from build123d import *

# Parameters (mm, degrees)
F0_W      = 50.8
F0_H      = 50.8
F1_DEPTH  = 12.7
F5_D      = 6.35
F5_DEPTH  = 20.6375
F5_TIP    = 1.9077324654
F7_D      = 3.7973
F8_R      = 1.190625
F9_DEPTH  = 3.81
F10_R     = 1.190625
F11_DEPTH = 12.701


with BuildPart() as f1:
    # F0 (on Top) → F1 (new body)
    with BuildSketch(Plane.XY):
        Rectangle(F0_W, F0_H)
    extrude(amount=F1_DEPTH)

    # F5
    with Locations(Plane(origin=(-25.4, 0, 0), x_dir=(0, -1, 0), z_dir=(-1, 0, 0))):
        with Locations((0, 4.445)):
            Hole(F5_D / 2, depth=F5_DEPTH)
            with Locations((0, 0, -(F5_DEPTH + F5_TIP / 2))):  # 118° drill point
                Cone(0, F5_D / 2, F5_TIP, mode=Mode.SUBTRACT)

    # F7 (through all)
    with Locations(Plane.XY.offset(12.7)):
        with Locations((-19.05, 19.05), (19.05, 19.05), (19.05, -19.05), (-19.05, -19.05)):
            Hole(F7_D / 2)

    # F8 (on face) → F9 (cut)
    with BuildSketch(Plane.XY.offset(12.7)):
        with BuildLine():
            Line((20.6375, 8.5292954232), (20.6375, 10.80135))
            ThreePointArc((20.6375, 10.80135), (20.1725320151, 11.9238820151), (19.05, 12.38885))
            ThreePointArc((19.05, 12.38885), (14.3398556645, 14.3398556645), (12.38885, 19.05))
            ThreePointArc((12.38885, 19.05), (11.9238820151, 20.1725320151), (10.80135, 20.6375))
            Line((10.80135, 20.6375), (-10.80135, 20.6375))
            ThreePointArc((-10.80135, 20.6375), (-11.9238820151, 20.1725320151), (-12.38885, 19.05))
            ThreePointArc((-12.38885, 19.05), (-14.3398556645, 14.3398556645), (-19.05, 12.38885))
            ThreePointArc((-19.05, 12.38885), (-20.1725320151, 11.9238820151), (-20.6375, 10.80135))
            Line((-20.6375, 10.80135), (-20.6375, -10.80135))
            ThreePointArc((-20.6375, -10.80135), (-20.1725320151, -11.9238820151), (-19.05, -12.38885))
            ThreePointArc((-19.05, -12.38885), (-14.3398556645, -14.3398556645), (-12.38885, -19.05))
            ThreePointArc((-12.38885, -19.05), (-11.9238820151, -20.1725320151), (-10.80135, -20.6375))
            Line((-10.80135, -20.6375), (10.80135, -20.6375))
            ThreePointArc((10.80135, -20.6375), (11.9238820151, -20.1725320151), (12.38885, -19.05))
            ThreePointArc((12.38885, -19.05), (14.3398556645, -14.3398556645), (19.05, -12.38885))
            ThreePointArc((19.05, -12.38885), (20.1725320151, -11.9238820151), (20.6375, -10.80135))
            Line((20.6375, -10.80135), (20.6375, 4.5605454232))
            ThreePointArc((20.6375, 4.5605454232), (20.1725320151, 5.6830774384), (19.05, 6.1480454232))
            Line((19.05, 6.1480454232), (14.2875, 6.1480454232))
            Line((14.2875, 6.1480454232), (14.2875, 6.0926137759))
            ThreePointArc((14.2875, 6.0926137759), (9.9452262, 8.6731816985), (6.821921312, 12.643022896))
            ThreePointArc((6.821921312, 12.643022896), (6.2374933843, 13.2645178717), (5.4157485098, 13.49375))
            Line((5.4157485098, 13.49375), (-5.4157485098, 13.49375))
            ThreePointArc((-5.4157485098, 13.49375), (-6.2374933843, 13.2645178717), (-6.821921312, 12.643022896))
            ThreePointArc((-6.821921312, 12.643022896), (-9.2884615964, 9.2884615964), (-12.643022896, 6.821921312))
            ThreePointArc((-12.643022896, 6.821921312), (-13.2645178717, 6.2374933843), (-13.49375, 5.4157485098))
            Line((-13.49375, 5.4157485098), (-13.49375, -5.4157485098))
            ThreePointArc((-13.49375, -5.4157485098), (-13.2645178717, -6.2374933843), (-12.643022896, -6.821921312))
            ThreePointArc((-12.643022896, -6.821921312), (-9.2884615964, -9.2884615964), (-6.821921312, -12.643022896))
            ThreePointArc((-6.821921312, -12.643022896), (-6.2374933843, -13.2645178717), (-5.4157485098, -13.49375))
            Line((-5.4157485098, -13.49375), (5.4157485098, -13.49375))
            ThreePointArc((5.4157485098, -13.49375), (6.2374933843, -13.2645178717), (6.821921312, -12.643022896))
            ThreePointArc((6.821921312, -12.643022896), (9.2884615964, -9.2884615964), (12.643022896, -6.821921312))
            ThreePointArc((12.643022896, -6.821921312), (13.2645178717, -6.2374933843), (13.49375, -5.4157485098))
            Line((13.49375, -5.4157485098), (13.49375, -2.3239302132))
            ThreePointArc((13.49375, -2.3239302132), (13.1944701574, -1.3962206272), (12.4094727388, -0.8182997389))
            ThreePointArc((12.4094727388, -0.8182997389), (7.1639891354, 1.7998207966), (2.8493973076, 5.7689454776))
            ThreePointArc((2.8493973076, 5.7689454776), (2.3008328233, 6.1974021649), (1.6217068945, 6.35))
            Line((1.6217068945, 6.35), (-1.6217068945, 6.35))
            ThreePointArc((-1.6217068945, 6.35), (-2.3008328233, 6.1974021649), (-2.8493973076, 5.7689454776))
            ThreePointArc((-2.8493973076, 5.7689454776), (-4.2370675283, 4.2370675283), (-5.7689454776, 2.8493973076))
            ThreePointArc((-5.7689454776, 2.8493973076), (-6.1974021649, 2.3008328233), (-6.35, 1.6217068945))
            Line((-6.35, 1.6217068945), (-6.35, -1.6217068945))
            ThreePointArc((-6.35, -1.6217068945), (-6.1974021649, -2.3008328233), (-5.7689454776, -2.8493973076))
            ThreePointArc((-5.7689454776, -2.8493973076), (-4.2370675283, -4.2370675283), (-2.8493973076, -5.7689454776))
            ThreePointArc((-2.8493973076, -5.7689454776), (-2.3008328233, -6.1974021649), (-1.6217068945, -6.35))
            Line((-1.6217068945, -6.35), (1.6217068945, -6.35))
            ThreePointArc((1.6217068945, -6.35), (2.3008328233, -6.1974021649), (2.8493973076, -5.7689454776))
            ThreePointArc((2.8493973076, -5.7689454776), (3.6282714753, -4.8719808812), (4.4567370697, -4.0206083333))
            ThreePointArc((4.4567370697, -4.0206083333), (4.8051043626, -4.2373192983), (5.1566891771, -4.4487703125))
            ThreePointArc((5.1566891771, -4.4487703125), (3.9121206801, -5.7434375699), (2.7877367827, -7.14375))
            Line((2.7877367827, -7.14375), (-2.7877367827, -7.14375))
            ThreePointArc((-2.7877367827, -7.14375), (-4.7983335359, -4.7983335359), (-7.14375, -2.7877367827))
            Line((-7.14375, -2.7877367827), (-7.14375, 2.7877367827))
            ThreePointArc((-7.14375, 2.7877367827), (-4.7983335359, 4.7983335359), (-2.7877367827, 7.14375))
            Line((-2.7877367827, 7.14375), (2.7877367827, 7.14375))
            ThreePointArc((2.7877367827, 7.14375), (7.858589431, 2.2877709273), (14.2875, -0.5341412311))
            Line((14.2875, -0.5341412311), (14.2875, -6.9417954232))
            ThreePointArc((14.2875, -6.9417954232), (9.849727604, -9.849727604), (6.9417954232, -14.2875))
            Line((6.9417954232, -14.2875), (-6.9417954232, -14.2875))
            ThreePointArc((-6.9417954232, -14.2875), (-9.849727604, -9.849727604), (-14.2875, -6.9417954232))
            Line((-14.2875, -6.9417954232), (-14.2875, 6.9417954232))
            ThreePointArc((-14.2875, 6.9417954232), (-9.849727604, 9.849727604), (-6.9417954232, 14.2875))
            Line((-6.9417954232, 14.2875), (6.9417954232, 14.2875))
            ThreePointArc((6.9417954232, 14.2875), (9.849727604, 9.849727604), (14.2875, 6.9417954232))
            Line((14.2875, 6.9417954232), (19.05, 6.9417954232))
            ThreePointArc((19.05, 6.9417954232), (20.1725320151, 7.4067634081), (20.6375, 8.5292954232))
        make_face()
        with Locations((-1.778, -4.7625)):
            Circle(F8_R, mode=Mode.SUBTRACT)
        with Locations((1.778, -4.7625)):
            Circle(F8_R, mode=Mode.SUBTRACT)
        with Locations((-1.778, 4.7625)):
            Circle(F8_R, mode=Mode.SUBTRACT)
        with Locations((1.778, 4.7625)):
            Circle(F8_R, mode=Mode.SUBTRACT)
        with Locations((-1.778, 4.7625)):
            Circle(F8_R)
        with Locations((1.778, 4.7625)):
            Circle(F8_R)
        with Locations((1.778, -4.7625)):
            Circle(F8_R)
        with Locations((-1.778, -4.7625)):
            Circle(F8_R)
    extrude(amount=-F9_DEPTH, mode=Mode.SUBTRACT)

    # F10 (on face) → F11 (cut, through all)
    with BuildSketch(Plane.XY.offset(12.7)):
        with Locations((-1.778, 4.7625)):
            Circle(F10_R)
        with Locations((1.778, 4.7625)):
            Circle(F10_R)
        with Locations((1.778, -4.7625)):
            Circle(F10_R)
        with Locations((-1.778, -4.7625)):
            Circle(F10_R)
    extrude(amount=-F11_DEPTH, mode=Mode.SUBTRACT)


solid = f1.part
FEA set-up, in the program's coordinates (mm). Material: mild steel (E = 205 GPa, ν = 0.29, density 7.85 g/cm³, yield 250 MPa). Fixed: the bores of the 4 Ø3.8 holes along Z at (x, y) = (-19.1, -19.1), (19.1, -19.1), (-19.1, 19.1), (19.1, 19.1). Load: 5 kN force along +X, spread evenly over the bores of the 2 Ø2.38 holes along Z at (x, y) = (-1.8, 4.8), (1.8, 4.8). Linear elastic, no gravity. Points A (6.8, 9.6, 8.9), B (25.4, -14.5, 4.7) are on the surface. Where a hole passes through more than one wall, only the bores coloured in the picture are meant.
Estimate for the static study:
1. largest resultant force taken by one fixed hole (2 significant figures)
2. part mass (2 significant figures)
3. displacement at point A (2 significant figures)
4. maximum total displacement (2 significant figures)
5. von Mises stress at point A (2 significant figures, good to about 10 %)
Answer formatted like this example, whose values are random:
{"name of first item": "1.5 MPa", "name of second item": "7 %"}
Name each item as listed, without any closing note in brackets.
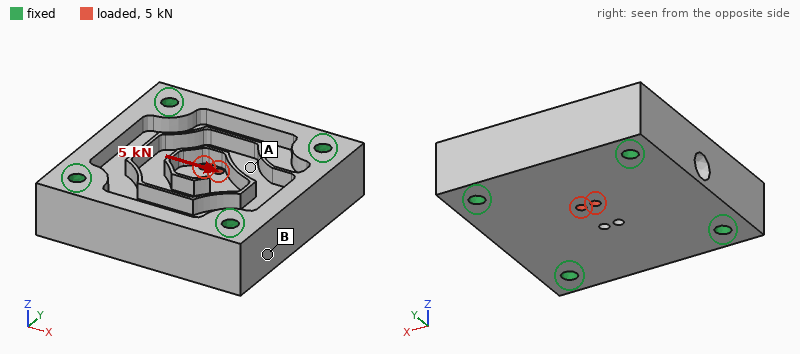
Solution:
{"largest resultant force taken by one fixed hole": "1.8 kN", "part mass": "210 g", "displacement at point A": "1.3 µm", "maximum total displacement": "3.4 µm", "von Mises stress at point A": "20 MPa"}
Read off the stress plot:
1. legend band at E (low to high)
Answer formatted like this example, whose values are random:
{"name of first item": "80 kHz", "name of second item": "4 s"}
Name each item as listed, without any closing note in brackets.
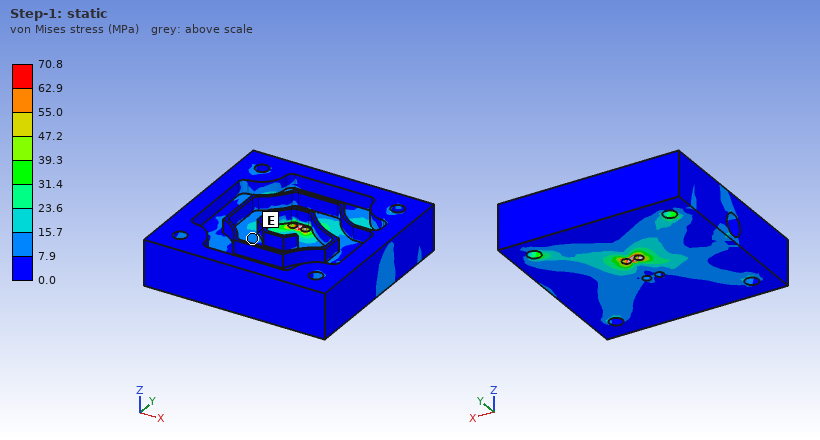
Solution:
{"legend band at E": "7.9 to 15.7 MPa"}
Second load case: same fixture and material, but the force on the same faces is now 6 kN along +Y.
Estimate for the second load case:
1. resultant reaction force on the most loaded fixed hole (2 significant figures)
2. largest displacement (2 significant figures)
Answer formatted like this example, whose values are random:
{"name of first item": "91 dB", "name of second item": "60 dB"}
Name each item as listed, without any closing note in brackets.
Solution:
{"resultant reaction force on the most loaded fixed hole": "1.9 kN", "largest displacement": "3.4 µm"}
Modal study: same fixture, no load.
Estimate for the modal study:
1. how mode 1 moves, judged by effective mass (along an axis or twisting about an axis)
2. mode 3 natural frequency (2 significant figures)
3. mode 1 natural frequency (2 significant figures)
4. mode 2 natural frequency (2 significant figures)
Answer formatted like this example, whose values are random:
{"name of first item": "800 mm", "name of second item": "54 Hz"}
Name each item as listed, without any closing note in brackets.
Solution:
{"how mode 1 moves, judged by effective mass": "along Z", "mode 3 natural frequency": "30 kHz", "mode 1 natural frequency": "20 kHz", "mode 2 natural frequency": "30 kHz"}
